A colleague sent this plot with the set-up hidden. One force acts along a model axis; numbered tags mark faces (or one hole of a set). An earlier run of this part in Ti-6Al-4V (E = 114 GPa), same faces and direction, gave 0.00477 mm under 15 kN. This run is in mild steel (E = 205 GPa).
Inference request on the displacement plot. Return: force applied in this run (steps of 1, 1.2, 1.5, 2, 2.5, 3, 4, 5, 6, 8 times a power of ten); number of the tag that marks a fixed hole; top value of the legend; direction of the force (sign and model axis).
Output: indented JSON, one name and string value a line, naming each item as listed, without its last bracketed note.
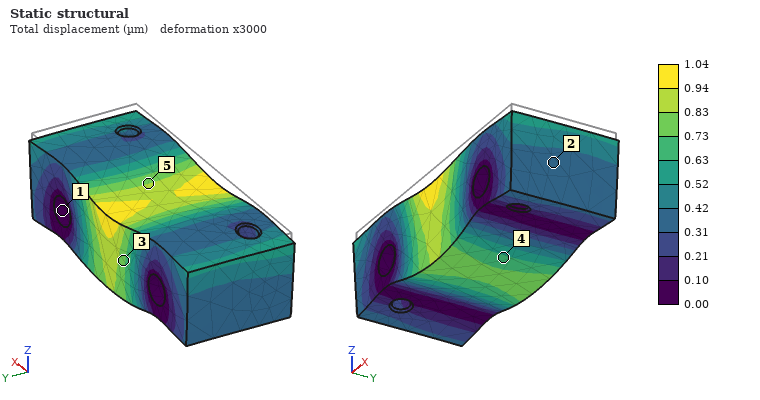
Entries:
{
  "force applied in this run": "6 kN",
  "number of the tag that marks a fixed hole": "1",
  "top value of the legend": "1.04 µm",
  "direction of the force": "-Z"
}
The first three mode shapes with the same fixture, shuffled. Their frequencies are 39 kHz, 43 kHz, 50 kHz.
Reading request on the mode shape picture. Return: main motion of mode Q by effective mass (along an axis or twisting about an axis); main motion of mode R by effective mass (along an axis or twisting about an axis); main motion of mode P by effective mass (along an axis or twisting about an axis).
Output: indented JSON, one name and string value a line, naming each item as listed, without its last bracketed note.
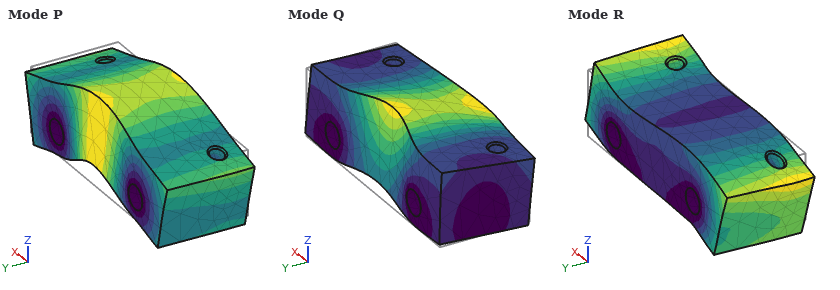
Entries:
{
  "main motion of mode Q by effective mass": "along Y",
  "main motion of mode R by effective mass": "along X",
  "main motion of mode P by effective mass": "along Z"
}
